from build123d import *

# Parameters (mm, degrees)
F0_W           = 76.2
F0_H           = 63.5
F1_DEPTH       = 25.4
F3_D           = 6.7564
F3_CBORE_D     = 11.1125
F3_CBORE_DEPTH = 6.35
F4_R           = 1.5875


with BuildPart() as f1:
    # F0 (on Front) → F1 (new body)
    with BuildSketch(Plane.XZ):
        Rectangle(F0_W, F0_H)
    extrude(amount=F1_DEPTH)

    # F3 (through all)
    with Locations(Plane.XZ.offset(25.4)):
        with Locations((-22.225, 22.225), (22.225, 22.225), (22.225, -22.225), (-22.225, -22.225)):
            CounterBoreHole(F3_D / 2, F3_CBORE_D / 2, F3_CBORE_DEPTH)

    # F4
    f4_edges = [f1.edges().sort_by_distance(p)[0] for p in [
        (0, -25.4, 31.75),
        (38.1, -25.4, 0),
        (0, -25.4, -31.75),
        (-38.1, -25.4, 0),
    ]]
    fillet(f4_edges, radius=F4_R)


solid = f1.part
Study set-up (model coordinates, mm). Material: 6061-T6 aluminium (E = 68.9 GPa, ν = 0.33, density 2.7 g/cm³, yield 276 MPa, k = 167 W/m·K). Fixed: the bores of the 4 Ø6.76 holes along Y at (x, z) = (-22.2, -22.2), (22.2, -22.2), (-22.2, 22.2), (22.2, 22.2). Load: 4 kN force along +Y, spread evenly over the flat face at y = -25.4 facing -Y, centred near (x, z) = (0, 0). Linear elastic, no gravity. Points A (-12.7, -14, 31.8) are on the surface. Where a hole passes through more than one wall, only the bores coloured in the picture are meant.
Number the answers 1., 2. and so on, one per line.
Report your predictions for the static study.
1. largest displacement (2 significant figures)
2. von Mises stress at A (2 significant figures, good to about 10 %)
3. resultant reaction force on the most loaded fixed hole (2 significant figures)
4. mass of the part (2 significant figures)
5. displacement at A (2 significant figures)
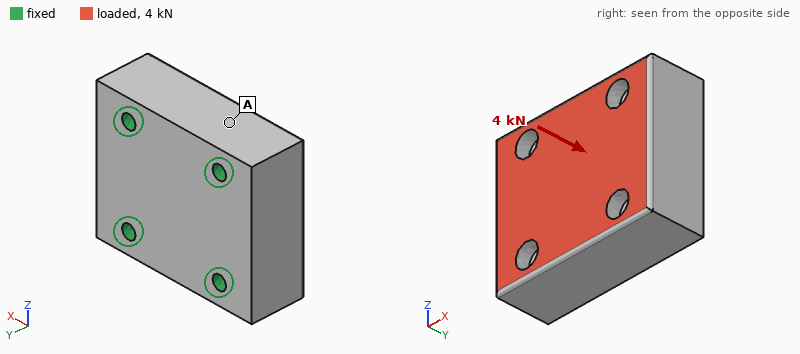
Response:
1. 1.1 µm
2. 1.2 MPa
3. 1.0 kN
4. 320 g
5. 0.39 µm
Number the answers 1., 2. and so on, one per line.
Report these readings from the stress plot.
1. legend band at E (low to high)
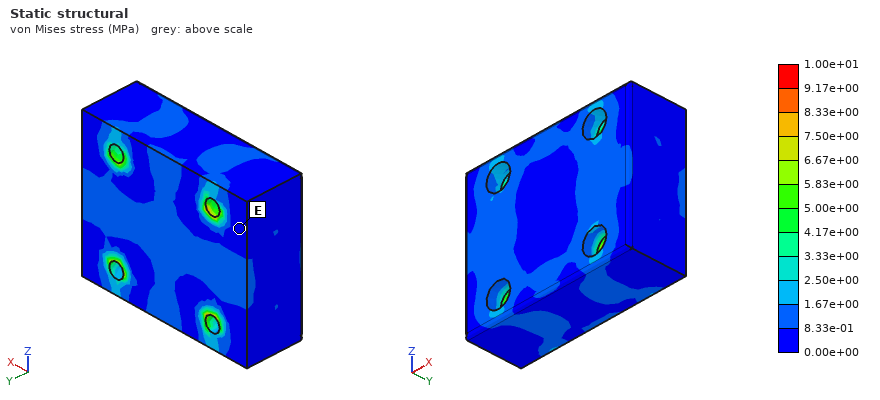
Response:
1. 0.00e+00 to 8.33e-01 MPa
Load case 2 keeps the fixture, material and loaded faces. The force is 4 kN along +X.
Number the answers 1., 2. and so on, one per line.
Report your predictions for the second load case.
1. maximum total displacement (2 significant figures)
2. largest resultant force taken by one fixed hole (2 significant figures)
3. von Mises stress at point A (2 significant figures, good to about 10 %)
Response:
1. 1.9 µm
2. 1.1 kN
3. 1.2 MPa
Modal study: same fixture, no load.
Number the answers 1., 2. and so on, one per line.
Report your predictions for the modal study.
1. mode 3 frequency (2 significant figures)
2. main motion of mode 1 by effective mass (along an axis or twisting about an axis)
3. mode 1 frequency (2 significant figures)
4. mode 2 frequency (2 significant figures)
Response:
1. 25 kHz
2. along Y
3. 21 kHz
4. 23 kHz
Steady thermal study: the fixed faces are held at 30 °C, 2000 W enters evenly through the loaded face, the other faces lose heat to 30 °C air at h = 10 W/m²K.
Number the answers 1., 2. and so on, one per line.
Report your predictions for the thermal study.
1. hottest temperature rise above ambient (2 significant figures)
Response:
1. 84 K
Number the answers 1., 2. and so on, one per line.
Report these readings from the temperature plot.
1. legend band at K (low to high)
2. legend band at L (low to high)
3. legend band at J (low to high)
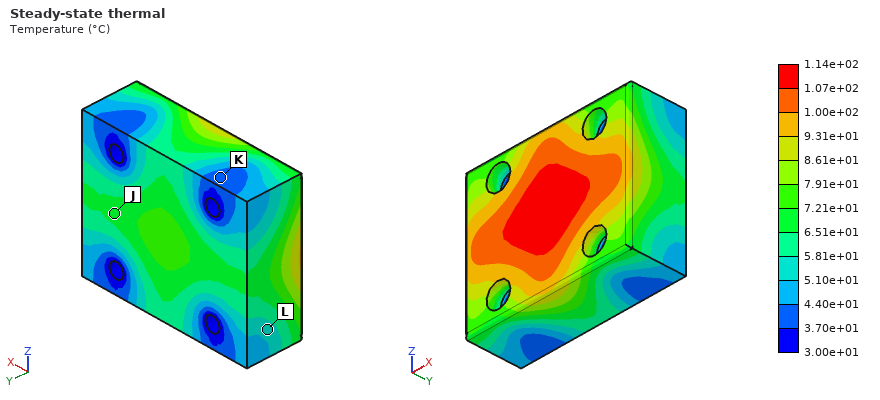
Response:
1. 3.70e+01 to 4.40e+01 °C
2. 5.10e+01 to 5.81e+01 °C
3. 6.51e+01 to 7.21e+01 °C
